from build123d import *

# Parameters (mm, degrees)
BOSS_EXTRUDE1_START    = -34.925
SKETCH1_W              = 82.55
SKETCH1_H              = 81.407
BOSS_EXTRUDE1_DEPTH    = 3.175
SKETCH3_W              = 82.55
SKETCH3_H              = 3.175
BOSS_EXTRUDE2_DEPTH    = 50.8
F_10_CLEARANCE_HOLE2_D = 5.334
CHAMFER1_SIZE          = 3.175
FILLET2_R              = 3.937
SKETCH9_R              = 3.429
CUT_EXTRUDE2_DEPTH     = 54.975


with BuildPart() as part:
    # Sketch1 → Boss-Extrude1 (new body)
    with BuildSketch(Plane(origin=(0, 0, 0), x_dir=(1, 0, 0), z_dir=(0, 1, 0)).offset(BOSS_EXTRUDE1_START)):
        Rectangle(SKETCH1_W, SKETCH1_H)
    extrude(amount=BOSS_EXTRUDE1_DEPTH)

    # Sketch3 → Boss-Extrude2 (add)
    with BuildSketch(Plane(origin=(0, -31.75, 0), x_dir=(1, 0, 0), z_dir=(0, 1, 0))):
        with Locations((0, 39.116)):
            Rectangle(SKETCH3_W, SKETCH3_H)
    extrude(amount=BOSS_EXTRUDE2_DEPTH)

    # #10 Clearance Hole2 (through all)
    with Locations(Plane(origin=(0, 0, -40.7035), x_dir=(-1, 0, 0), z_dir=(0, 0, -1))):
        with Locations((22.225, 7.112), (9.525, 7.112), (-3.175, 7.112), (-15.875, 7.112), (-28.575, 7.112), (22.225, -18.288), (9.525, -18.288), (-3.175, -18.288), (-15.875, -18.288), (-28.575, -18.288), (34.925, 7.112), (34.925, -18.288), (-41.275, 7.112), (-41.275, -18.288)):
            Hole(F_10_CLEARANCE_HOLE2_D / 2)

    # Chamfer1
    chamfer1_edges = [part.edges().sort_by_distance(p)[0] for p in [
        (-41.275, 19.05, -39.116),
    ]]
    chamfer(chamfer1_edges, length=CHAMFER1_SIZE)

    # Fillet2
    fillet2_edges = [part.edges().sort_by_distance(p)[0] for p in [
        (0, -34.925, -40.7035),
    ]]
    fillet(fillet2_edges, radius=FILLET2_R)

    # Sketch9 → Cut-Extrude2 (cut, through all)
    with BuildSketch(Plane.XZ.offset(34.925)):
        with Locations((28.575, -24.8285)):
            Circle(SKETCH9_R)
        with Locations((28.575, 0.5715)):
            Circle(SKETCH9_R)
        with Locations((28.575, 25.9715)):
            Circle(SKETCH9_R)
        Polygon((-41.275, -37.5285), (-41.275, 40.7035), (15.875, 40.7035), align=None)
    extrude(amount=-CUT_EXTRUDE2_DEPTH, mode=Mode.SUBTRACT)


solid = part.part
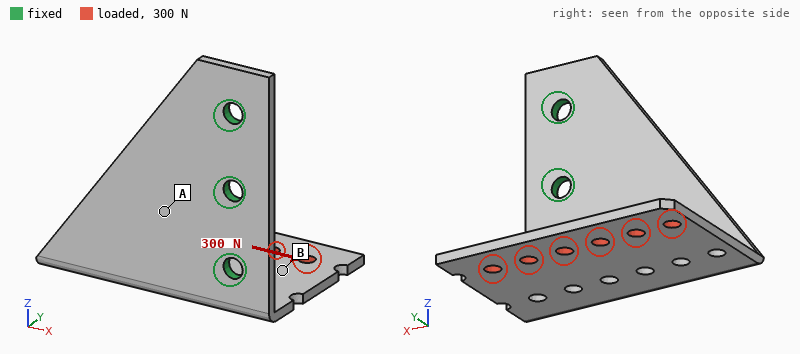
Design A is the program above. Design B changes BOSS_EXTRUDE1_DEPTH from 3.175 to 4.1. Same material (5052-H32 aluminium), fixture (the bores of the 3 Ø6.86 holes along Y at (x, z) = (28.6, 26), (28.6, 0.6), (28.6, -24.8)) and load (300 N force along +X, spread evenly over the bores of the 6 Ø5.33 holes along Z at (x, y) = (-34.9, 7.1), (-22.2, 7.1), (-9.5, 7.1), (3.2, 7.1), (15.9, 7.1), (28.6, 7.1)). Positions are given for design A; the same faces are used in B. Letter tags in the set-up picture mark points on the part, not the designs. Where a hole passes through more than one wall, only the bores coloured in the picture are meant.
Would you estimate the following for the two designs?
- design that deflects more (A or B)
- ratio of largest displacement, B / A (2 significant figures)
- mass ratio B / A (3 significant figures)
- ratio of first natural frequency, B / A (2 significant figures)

A
0.53
1.15
1.3
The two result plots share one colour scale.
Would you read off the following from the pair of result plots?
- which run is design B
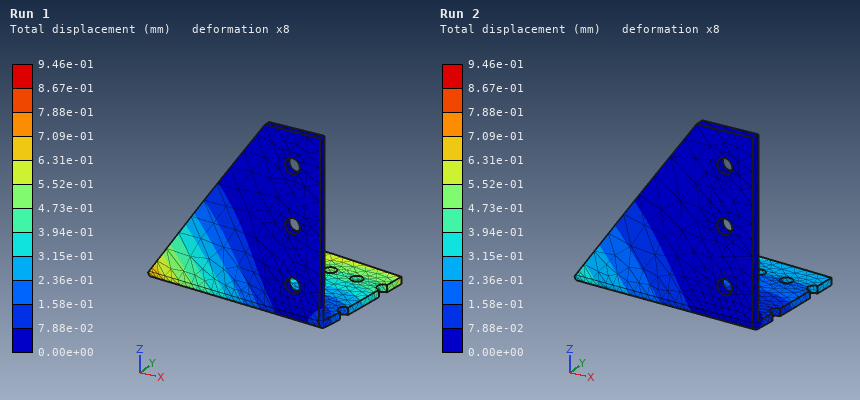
Run 2
